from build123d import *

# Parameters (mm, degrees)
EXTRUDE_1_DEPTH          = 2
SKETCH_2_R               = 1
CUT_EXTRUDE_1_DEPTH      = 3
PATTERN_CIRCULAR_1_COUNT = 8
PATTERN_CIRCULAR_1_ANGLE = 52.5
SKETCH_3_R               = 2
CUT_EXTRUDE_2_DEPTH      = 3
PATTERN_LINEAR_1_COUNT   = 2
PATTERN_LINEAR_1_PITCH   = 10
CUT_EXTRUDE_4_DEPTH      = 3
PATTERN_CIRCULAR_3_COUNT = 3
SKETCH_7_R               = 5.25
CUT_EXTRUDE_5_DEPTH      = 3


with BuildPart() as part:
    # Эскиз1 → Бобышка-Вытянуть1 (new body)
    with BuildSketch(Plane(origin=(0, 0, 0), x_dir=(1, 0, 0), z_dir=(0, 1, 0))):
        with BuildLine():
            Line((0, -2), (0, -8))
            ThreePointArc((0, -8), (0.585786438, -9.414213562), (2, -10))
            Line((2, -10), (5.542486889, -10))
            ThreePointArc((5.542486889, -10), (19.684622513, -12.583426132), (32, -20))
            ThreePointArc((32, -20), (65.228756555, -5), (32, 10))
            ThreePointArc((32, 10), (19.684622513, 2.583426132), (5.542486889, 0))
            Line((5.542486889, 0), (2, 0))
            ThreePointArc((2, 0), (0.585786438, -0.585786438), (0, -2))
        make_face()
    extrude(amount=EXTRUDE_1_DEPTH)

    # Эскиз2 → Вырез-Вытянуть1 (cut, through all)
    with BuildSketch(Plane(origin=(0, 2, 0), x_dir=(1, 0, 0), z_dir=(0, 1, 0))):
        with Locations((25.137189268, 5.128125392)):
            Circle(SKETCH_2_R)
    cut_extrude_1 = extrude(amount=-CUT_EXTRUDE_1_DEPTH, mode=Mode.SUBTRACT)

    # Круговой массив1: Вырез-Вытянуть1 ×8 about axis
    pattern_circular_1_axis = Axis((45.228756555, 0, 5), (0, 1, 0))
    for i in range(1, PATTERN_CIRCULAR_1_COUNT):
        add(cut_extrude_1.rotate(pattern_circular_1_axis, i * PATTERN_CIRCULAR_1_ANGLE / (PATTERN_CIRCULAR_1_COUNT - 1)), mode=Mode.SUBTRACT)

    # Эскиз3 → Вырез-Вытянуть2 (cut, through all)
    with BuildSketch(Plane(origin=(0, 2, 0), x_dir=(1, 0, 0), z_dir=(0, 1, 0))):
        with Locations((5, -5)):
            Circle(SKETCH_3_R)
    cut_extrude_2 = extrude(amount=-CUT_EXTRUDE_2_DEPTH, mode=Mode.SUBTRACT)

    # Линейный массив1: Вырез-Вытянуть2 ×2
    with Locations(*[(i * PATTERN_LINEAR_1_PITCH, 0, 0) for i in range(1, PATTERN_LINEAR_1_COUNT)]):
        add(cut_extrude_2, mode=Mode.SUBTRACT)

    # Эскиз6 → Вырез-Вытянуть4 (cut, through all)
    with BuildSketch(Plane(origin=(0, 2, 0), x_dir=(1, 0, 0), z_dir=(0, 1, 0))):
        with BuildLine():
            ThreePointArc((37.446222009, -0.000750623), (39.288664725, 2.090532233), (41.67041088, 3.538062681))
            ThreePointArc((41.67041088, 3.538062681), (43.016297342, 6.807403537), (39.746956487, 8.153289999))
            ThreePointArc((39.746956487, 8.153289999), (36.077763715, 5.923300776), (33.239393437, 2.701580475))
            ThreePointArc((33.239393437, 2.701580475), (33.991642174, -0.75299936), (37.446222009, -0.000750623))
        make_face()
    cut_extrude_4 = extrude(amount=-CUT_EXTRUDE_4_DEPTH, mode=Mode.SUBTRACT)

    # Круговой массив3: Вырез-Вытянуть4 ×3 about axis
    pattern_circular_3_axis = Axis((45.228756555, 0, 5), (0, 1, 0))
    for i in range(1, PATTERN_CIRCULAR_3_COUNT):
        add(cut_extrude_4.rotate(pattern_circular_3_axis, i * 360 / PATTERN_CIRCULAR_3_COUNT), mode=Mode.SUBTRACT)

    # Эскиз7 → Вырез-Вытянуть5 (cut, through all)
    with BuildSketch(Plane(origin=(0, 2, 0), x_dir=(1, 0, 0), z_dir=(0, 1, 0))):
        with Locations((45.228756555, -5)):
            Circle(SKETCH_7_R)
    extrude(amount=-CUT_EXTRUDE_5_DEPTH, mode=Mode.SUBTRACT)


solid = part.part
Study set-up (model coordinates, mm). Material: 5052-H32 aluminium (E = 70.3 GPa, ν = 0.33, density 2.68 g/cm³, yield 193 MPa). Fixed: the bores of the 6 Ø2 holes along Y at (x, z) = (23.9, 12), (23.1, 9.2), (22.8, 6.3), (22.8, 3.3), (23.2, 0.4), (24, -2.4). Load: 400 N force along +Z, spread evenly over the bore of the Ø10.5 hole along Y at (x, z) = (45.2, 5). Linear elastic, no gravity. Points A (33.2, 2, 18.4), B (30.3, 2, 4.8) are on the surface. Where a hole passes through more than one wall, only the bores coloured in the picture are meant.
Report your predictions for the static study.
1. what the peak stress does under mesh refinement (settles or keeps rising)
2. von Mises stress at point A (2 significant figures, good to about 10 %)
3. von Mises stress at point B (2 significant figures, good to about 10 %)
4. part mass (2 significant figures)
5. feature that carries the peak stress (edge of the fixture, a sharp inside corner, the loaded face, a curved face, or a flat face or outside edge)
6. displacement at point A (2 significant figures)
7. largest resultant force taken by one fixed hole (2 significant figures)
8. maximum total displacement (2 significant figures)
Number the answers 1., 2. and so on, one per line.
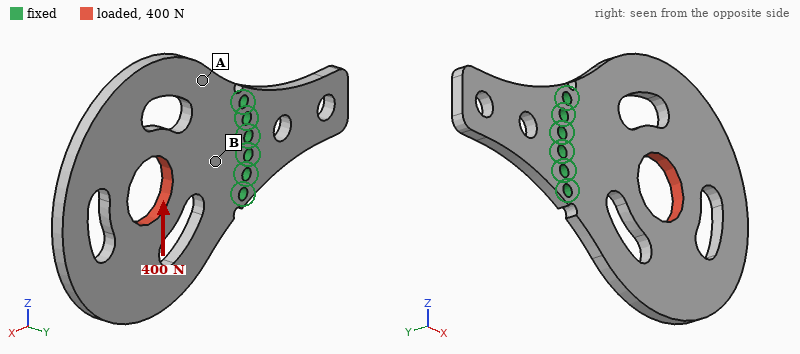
1. keeps rising
2. 13 MPa
3. 32 MPa
4. 7.0 g
5. edge of the fixture
6. 16 µm
7. 500 N
8. 58 µm
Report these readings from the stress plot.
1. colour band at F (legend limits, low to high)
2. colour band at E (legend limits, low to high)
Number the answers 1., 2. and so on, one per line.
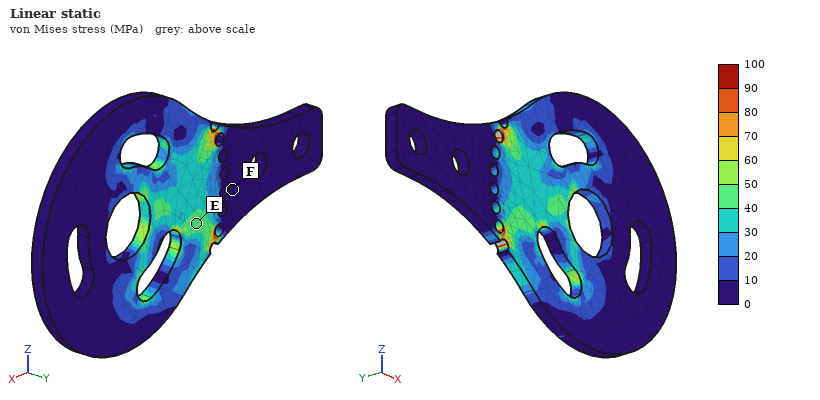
1. 0 to 10 MPa
2. 40 to 50 MPa
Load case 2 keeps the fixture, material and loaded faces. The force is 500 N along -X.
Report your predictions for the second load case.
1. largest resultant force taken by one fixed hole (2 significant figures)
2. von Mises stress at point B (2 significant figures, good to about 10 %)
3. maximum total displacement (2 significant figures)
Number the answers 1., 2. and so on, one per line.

1. 130 N
2. 16 MPa
3. 11 µm
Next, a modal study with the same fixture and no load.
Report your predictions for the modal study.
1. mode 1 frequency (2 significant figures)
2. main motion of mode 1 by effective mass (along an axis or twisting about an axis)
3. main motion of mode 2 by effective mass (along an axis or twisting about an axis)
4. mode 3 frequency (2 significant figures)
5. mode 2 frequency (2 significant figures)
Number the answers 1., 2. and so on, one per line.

1. 940 Hz
2. along Y
3. twisting about X
4. 4000 Hz
5. 2200 Hz
